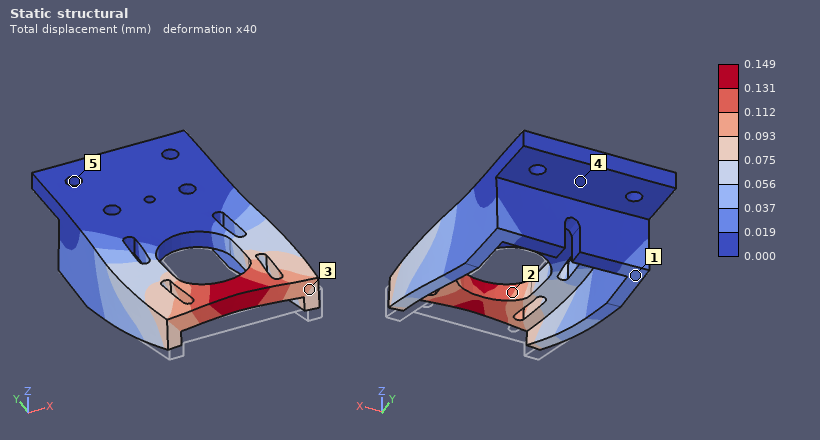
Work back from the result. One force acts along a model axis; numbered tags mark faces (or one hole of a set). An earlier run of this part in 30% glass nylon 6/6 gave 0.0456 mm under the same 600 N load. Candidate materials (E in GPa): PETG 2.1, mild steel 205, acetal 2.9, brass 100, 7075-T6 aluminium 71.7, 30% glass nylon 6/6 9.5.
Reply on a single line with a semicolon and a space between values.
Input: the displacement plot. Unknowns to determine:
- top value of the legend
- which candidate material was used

0.149 mm; acetal
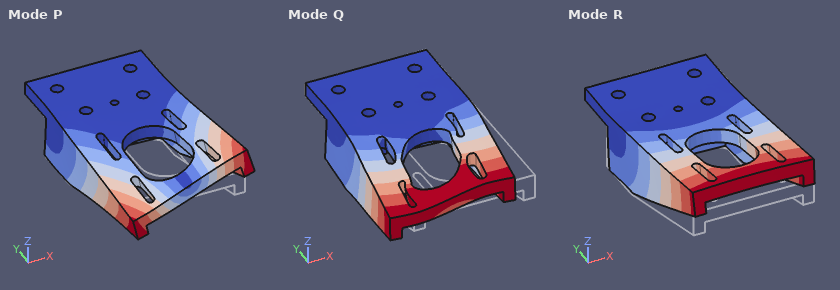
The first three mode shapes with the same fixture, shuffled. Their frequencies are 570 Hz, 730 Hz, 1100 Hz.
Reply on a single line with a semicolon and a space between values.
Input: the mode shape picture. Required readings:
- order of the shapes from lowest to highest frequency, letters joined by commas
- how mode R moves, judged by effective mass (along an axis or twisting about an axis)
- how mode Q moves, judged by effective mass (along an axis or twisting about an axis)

R, P, Q; along Z; along X
